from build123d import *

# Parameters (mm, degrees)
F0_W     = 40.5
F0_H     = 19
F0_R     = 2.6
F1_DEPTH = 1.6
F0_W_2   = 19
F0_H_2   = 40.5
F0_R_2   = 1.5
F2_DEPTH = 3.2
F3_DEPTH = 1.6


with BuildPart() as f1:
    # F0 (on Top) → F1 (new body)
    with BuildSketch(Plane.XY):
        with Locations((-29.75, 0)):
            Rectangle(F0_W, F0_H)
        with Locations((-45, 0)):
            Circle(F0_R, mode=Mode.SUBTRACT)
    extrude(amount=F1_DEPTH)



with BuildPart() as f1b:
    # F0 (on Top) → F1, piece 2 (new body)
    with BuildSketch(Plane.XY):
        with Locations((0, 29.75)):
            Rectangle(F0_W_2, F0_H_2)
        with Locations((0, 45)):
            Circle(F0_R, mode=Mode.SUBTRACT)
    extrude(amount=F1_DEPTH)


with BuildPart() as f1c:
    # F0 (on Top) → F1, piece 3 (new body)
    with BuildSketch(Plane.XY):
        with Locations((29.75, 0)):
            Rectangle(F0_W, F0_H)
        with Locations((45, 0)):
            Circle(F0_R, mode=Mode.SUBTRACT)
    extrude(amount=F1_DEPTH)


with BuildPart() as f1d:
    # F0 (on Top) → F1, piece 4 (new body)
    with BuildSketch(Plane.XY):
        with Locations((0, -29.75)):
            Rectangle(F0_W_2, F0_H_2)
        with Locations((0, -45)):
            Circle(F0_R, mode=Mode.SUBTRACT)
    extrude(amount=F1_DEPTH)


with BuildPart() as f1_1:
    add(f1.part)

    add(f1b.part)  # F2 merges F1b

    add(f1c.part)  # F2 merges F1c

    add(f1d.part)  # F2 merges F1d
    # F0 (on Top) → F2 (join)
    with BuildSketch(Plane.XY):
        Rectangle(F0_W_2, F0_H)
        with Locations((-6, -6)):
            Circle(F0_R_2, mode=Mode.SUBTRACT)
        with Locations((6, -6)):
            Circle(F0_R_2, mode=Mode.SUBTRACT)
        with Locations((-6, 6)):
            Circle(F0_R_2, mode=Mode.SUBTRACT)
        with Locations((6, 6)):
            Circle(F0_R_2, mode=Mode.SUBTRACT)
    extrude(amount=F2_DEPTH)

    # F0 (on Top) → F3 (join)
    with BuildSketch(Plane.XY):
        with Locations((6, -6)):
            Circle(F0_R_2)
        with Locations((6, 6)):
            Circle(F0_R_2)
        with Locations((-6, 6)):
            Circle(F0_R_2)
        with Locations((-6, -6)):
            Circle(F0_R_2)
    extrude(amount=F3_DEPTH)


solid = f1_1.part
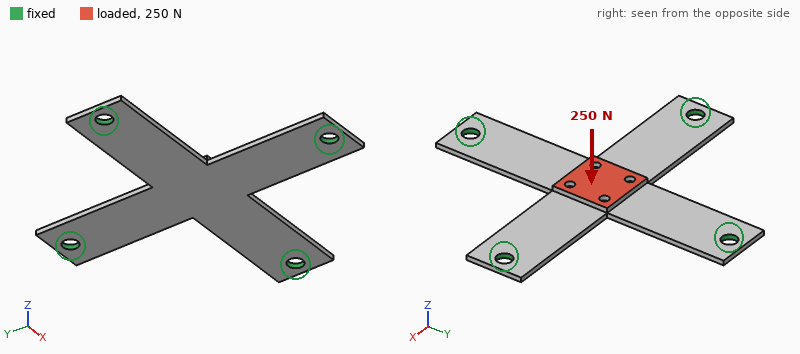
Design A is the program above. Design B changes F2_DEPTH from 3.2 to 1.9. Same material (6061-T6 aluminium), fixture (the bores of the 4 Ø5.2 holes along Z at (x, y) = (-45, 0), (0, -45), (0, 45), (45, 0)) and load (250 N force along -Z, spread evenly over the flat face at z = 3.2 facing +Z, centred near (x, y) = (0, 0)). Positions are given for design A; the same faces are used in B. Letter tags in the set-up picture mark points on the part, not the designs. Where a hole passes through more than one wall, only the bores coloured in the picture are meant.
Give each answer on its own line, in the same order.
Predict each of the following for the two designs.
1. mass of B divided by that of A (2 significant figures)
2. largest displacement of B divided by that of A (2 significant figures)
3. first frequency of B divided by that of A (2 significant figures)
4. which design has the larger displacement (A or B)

0.93
1.2
1.0
B
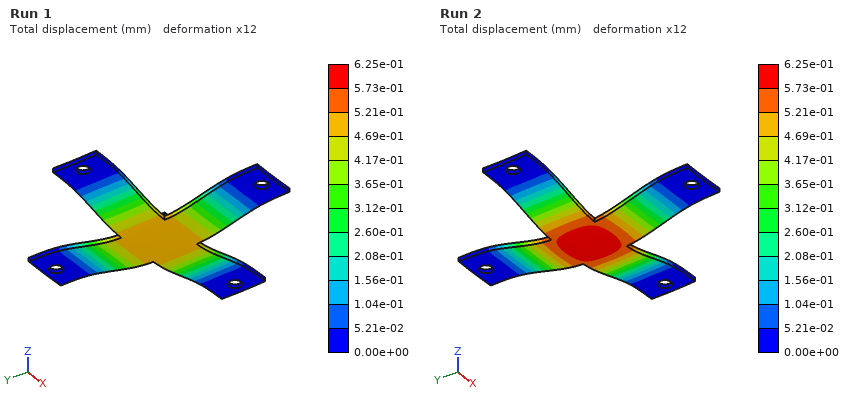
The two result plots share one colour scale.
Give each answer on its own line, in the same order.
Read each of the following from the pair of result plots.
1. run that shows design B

Run 2
